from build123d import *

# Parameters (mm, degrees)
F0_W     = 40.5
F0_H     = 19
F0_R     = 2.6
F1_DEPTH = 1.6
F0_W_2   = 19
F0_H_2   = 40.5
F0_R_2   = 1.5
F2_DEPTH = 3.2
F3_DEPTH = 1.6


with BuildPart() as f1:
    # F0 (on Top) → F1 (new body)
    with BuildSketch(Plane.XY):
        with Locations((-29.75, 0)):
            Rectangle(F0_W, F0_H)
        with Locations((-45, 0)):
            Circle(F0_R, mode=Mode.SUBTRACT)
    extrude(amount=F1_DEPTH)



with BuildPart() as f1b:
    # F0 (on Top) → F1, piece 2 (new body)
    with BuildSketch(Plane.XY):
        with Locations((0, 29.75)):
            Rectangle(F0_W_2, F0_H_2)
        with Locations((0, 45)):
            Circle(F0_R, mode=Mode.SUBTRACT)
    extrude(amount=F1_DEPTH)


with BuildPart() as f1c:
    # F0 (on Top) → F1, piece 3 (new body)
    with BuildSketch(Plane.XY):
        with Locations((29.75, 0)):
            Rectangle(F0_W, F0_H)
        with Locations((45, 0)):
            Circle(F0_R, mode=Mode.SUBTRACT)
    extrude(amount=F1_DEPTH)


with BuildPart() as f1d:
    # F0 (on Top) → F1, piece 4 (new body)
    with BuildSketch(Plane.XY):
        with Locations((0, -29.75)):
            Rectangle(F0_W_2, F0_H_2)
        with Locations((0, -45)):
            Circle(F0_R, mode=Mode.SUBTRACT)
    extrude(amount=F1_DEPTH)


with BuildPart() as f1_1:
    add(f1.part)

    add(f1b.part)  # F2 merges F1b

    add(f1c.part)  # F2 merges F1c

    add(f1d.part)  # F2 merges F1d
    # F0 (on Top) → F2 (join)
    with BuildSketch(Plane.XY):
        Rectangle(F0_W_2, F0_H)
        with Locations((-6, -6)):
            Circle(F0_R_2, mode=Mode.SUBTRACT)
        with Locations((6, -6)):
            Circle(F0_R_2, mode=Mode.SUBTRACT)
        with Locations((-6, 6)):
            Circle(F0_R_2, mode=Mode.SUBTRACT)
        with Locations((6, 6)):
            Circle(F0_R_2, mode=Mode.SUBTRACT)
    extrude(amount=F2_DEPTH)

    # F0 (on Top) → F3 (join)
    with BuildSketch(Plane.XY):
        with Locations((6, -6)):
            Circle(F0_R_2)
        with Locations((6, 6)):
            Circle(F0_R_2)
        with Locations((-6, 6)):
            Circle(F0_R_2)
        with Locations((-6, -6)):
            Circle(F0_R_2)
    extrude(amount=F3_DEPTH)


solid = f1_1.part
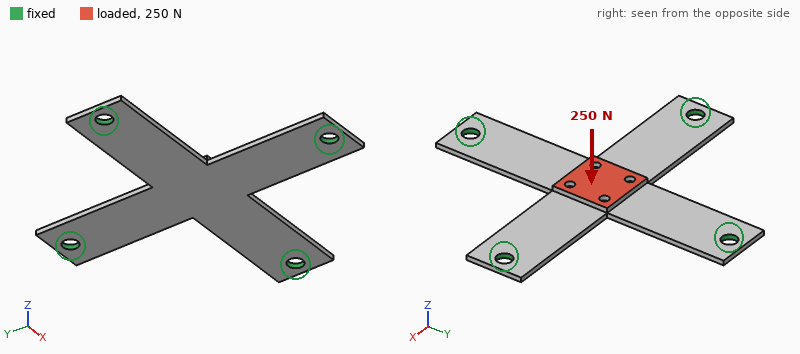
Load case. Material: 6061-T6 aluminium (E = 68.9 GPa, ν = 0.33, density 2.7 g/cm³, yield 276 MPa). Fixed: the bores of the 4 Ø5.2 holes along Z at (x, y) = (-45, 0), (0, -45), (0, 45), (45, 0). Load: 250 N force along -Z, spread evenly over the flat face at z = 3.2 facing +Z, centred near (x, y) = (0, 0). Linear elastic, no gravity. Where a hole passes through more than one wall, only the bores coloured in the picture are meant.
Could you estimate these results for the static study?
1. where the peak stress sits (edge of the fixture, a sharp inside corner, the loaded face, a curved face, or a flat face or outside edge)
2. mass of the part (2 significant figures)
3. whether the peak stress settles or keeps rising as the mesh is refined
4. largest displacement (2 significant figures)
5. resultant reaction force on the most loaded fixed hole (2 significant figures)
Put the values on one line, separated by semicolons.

edge of the fixture; 16 g; keeps rising; 0.50 mm; 86 N
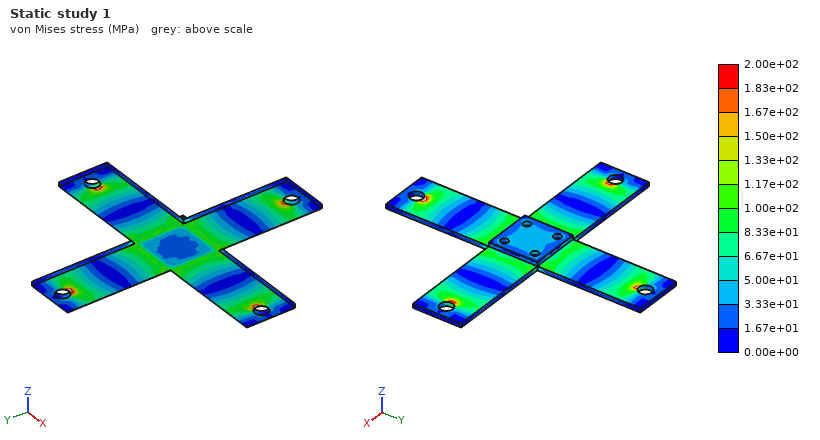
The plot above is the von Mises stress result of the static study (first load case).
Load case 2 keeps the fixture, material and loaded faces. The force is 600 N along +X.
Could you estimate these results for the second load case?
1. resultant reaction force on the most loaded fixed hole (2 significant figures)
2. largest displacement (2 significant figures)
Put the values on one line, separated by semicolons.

280 N; 73 µm
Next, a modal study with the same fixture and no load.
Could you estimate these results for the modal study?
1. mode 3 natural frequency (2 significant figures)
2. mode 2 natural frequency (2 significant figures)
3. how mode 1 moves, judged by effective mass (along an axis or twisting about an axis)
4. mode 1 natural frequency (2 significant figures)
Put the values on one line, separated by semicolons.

3100 Hz; 3100 Hz; along Z; 1400 Hz
